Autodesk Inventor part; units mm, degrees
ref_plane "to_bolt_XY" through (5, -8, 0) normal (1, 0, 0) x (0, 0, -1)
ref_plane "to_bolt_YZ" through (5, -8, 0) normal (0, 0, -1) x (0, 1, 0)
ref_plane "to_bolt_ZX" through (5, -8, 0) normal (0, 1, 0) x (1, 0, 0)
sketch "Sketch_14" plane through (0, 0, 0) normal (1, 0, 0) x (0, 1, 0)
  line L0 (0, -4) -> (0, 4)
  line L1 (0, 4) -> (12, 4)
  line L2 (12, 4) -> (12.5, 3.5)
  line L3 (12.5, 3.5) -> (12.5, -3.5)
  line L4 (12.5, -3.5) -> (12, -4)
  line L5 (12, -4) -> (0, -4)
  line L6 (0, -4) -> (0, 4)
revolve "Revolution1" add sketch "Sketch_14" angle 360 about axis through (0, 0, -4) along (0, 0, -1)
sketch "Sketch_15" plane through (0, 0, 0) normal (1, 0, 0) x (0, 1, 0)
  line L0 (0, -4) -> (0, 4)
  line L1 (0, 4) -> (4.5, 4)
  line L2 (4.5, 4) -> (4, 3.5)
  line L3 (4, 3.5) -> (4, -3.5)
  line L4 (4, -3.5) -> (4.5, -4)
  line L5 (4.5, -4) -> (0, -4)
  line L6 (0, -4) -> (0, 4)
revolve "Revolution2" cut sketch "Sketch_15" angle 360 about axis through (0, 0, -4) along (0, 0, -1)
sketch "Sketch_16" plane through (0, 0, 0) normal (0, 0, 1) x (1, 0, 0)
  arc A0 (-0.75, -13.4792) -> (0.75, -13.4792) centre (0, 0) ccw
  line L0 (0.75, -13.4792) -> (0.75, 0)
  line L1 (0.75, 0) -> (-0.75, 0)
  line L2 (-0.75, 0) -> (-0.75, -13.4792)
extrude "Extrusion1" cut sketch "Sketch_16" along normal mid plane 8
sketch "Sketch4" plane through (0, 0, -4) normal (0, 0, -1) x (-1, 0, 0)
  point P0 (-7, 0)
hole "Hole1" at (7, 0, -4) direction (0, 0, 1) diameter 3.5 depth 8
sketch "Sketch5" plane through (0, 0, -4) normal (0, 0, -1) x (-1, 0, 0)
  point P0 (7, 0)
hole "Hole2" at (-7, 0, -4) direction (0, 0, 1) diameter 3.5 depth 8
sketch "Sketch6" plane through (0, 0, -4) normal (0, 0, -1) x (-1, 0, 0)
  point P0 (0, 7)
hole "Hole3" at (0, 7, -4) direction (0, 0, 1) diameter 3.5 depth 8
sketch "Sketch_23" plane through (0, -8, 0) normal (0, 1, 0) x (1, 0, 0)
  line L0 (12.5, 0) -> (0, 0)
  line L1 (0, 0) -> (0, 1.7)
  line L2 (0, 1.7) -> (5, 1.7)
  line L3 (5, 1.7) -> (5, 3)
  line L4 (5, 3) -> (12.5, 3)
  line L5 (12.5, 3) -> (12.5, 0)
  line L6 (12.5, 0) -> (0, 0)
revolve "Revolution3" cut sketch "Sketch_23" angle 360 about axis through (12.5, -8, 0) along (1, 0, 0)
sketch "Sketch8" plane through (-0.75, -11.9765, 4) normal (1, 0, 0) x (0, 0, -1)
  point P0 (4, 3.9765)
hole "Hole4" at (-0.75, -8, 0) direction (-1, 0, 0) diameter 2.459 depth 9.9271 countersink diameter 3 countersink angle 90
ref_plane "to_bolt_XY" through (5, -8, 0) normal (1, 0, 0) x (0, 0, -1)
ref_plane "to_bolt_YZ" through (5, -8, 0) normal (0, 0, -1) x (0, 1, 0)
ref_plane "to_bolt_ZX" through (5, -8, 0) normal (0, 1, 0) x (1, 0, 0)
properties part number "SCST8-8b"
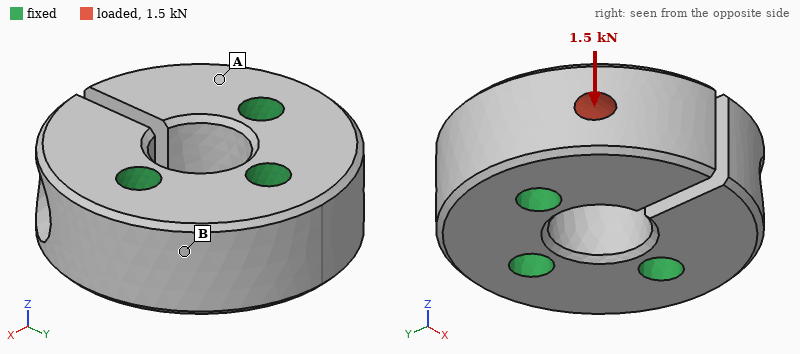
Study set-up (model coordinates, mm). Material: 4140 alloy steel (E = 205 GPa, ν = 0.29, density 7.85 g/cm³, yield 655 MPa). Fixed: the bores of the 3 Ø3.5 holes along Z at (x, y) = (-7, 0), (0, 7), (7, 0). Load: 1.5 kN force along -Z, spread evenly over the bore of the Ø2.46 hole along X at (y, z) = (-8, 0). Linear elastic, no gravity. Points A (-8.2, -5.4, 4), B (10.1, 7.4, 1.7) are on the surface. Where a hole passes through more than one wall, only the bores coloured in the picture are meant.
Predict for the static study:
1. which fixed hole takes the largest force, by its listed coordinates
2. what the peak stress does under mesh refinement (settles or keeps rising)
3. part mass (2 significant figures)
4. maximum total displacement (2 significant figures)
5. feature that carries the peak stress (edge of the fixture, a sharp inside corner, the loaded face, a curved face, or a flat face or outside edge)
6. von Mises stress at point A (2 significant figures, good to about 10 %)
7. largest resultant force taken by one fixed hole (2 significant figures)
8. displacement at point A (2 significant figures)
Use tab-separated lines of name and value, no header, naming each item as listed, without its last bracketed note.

which fixed hole takes the largest force, by its listed coordinates	(-7, 0)
what the peak stress does under mesh refinement	keeps rising
part mass	23 g
maximum total displacement	9.6 µm
feature that carries the peak stress	edge of the fixture
von Mises stress at point A	57 MPa
largest resultant force taken by one fixed hole	1.5 kN
displacement at point A	3.2 µm
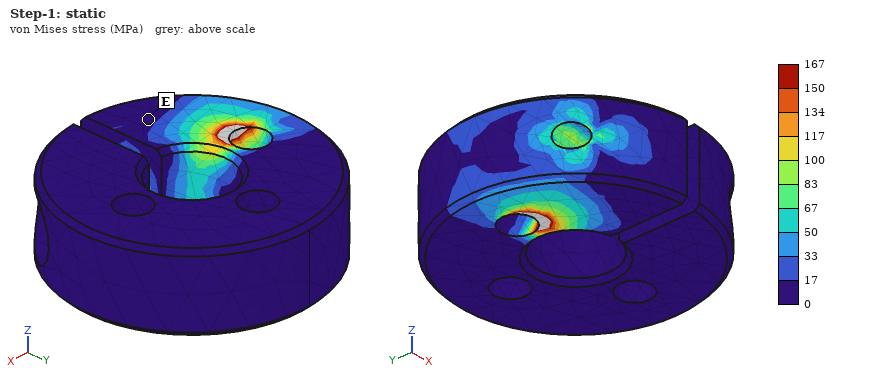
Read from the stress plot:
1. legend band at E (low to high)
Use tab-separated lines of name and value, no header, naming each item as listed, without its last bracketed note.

legend band at E	0 to 17 MPa
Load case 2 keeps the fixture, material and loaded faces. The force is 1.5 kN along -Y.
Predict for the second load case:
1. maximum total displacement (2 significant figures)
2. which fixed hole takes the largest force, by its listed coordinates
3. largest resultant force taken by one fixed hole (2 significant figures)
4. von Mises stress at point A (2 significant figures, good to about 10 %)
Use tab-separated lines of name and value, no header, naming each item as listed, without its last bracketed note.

maximum total displacement	4.0 µm
which fixed hole takes the largest force, by its listed coordinates	(-7, 0)
largest resultant force taken by one fixed hole	1.5 kN
von Mises stress at point A	16 MPa
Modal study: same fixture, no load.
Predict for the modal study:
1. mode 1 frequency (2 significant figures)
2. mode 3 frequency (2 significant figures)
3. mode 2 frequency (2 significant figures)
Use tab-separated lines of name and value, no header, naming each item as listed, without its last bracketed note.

mode 1 frequency	35 kHz
mode 3 frequency	36 kHz
mode 2 frequency	35 kHz
